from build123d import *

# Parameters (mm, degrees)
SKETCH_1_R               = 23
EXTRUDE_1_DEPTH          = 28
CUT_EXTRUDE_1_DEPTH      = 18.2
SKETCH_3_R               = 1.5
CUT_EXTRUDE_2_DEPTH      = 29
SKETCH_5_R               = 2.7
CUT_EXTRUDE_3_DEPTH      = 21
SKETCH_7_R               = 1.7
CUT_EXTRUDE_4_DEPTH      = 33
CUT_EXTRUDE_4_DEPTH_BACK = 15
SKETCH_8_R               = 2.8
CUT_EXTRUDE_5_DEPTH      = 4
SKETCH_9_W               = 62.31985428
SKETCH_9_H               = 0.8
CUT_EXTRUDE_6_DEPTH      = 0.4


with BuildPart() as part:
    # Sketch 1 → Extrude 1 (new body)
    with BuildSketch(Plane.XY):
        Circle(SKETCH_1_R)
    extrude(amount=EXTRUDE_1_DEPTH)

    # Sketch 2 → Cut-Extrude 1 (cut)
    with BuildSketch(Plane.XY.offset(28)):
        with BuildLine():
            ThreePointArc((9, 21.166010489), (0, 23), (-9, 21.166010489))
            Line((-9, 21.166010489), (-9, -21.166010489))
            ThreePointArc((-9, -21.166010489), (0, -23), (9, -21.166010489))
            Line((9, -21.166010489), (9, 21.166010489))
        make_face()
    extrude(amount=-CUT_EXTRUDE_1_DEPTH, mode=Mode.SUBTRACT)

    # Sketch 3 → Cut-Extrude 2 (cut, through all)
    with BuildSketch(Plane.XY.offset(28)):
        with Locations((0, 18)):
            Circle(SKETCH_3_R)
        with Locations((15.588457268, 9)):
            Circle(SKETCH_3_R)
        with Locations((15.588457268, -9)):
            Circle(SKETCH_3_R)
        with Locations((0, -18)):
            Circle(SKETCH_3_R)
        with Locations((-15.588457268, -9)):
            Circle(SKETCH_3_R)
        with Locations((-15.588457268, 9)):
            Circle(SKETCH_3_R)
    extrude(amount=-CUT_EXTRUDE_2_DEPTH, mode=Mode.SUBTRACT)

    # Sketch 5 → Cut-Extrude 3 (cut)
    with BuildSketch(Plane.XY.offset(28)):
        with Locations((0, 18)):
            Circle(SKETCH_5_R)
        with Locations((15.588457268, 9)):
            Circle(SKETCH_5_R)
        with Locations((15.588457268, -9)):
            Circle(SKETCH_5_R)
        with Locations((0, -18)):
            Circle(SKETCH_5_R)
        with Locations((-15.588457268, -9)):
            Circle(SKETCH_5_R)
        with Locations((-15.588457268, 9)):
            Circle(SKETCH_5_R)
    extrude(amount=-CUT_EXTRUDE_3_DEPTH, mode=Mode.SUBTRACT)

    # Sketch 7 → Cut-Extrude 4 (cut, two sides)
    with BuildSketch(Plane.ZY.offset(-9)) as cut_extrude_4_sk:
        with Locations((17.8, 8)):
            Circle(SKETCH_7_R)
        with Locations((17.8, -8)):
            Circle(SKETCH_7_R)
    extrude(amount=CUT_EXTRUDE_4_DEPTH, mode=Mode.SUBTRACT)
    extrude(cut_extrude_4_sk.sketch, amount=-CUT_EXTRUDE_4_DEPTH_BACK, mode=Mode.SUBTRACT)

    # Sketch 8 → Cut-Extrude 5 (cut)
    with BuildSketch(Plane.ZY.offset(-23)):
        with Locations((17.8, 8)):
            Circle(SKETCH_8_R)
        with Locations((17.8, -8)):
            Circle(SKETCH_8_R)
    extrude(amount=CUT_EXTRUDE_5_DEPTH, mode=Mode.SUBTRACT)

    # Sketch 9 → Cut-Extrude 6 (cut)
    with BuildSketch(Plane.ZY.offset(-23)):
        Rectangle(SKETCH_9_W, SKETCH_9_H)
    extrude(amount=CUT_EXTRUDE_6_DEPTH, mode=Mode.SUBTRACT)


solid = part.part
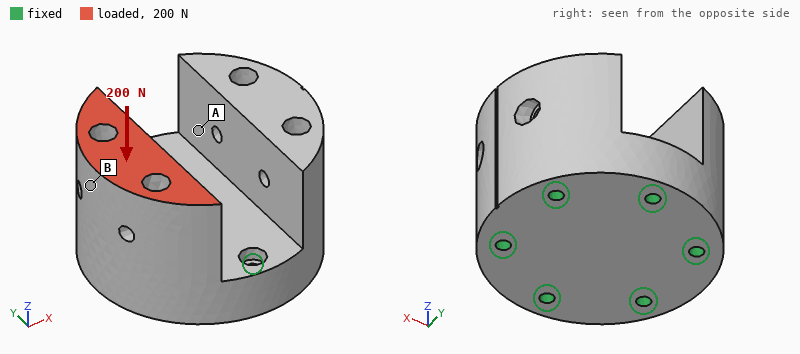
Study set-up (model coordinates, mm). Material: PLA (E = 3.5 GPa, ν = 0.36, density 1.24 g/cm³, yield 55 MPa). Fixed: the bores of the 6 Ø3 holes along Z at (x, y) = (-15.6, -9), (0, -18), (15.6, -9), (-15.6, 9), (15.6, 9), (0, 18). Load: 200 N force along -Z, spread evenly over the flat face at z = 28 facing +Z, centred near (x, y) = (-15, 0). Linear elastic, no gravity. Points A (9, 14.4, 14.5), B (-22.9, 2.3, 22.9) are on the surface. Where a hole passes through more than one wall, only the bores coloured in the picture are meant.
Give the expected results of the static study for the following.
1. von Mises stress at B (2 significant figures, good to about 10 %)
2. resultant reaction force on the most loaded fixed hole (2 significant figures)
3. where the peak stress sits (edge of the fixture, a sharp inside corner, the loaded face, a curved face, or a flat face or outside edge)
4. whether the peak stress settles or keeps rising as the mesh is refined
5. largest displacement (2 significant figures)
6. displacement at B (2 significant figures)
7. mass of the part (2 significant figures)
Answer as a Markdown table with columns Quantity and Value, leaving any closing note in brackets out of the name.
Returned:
| Quantity | Value |
|---|---|
| von Mises stress at B | 0.56 MPa |
| resultant reaction force on the most loaded fixed hole | 87 N |
| where the peak stress sits | edge of the fixture |
| whether the peak stress settles or keeps rising as the mesh is refined | keeps rising |
| largest displacement | 7.5 µm |
| displacement at B | 6.5 µm |
| mass of the part | 36 g |
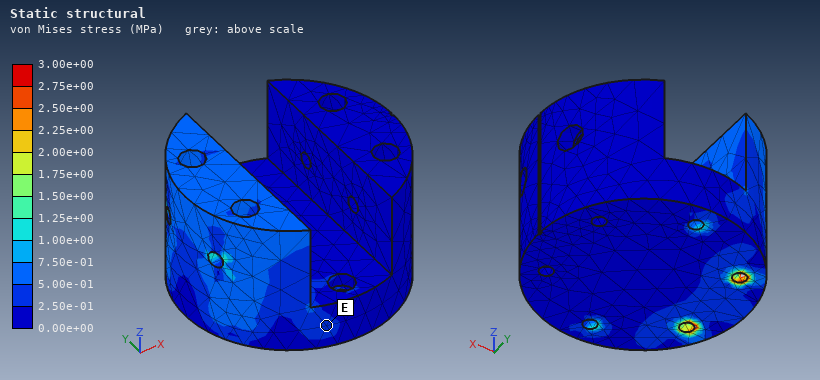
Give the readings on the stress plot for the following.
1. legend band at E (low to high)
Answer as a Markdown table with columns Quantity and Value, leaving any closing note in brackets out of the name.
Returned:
| Quantity | Value |
|---|---|
| legend band at E | 2.50e-01 to 5.00e-01 MPa |
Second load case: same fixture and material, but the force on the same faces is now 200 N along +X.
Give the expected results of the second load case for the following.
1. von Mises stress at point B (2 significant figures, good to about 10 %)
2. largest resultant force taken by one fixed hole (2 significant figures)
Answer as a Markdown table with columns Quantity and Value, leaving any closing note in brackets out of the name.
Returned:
| Quantity | Value |
|---|---|
| von Mises stress at point B | 1.6 MPa |
| largest resultant force taken by one fixed hole | 110 N |
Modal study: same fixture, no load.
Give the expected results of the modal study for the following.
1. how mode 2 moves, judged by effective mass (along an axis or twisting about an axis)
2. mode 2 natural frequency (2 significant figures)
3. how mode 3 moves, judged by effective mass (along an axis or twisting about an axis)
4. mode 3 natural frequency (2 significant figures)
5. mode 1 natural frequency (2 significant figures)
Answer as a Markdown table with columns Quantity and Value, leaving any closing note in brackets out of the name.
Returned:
| Quantity | Value |
|---|---|
| how mode 2 moves, judged by effective mass | along X |
| mode 2 natural frequency | 4500 Hz |
| how mode 3 moves, judged by effective mass | along Y |
| mode 3 natural frequency | 6300 Hz |
| mode 1 natural frequency | 4300 Hz |
